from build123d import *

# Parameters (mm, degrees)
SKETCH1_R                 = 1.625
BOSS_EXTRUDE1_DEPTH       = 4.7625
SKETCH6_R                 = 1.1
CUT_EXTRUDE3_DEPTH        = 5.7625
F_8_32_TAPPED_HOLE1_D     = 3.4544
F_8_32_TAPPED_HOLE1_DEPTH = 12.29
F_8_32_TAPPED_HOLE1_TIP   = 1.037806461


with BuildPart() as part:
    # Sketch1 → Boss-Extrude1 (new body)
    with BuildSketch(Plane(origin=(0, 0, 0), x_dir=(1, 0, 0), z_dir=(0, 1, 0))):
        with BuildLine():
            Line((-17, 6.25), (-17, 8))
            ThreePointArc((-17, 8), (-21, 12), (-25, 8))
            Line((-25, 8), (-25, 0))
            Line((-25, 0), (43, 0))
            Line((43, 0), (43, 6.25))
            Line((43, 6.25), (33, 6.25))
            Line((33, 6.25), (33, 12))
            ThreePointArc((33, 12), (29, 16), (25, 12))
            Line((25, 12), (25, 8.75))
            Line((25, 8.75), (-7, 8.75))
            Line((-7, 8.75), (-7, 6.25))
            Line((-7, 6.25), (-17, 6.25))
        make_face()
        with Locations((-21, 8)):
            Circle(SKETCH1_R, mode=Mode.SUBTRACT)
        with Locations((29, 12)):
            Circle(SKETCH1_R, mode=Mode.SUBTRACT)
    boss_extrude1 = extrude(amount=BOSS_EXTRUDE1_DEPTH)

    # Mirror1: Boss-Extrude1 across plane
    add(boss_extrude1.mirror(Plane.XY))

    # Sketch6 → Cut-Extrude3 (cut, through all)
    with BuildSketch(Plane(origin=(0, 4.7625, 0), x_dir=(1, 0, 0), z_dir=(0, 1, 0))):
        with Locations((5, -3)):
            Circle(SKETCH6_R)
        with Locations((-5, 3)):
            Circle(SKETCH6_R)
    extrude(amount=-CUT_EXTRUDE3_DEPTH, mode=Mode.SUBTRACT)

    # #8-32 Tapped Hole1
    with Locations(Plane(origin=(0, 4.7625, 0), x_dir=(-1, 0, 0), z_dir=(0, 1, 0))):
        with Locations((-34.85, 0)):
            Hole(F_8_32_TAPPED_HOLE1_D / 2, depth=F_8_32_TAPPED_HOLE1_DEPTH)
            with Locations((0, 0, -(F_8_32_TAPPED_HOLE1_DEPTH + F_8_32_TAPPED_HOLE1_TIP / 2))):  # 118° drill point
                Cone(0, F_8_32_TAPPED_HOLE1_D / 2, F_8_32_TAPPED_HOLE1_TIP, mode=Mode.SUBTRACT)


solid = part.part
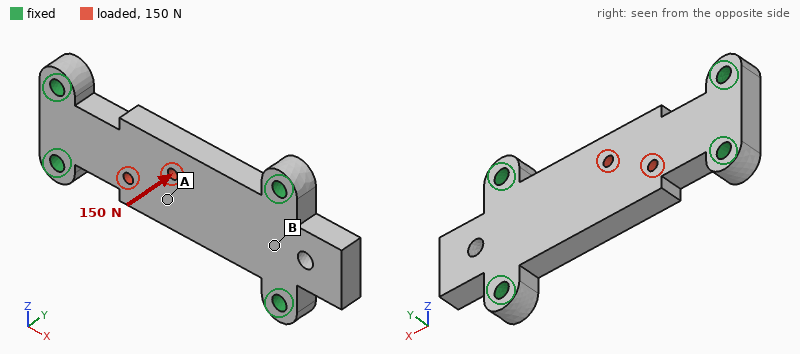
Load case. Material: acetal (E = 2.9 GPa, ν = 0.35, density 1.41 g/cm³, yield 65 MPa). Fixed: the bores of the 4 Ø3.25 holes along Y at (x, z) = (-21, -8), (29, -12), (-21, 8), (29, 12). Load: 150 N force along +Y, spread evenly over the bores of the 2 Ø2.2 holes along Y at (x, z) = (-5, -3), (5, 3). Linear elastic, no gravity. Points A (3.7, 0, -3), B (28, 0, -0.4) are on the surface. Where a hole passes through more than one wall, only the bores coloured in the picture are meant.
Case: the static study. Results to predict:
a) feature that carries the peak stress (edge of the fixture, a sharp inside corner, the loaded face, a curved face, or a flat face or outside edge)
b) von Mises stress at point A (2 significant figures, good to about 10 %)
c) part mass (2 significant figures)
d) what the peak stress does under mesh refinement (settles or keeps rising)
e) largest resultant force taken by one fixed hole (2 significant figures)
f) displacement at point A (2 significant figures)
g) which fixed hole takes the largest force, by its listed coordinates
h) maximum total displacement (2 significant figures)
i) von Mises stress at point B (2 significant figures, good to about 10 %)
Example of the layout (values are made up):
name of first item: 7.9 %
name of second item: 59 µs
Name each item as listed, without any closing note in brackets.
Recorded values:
feature that carries the peak stress: edge of the fixture
von Mises stress at point A: 9.8 MPa
part mass: 7.9 g
what the peak stress does under mesh refinement: keeps rising
largest resultant force taken by one fixed hole: 50 N
displacement at point A: 0.26 mm
which fixed hole takes the largest force, by its listed coordinates: (-21, -8)
maximum total displacement: 0.29 mm
von Mises stress at point B: 3.4 MPa
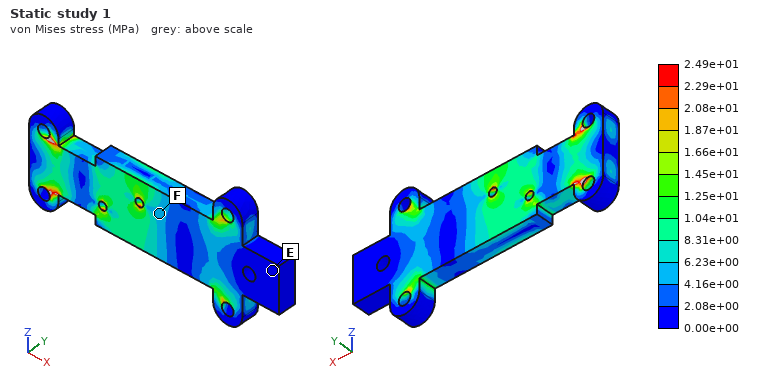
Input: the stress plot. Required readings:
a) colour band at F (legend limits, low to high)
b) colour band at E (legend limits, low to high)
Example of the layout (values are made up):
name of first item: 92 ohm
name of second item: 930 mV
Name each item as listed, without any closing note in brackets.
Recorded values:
colour band at F: 4.16e+00 to 6.23e+00 MPa
colour band at E: 0.00e+00 to 2.08e+00 MPa
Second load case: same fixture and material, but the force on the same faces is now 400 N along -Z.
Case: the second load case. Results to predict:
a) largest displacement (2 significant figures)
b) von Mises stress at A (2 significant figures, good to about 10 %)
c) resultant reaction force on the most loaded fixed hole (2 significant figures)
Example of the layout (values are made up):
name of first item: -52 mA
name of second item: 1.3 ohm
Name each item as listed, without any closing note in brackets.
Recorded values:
largest displacement: 0.10 mm
von Mises stress at A: 3.4 MPa
resultant reaction force on the most loaded fixed hole: 180 N
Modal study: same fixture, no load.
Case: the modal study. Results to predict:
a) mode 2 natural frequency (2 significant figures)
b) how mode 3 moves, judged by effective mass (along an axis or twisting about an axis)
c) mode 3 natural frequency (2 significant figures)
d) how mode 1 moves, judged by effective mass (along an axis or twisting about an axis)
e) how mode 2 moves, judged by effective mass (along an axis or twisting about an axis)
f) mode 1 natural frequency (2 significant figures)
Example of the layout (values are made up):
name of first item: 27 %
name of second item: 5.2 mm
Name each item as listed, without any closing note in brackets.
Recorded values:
mode 2 natural frequency: 3900 Hz
how mode 3 moves, judged by effective mass: twisting about X
mode 3 natural frequency: 4600 Hz
how mode 1 moves, judged by effective mass: along Y
how mode 2 moves, judged by effective mass: along Y
mode 1 natural frequency: 2200 Hz
